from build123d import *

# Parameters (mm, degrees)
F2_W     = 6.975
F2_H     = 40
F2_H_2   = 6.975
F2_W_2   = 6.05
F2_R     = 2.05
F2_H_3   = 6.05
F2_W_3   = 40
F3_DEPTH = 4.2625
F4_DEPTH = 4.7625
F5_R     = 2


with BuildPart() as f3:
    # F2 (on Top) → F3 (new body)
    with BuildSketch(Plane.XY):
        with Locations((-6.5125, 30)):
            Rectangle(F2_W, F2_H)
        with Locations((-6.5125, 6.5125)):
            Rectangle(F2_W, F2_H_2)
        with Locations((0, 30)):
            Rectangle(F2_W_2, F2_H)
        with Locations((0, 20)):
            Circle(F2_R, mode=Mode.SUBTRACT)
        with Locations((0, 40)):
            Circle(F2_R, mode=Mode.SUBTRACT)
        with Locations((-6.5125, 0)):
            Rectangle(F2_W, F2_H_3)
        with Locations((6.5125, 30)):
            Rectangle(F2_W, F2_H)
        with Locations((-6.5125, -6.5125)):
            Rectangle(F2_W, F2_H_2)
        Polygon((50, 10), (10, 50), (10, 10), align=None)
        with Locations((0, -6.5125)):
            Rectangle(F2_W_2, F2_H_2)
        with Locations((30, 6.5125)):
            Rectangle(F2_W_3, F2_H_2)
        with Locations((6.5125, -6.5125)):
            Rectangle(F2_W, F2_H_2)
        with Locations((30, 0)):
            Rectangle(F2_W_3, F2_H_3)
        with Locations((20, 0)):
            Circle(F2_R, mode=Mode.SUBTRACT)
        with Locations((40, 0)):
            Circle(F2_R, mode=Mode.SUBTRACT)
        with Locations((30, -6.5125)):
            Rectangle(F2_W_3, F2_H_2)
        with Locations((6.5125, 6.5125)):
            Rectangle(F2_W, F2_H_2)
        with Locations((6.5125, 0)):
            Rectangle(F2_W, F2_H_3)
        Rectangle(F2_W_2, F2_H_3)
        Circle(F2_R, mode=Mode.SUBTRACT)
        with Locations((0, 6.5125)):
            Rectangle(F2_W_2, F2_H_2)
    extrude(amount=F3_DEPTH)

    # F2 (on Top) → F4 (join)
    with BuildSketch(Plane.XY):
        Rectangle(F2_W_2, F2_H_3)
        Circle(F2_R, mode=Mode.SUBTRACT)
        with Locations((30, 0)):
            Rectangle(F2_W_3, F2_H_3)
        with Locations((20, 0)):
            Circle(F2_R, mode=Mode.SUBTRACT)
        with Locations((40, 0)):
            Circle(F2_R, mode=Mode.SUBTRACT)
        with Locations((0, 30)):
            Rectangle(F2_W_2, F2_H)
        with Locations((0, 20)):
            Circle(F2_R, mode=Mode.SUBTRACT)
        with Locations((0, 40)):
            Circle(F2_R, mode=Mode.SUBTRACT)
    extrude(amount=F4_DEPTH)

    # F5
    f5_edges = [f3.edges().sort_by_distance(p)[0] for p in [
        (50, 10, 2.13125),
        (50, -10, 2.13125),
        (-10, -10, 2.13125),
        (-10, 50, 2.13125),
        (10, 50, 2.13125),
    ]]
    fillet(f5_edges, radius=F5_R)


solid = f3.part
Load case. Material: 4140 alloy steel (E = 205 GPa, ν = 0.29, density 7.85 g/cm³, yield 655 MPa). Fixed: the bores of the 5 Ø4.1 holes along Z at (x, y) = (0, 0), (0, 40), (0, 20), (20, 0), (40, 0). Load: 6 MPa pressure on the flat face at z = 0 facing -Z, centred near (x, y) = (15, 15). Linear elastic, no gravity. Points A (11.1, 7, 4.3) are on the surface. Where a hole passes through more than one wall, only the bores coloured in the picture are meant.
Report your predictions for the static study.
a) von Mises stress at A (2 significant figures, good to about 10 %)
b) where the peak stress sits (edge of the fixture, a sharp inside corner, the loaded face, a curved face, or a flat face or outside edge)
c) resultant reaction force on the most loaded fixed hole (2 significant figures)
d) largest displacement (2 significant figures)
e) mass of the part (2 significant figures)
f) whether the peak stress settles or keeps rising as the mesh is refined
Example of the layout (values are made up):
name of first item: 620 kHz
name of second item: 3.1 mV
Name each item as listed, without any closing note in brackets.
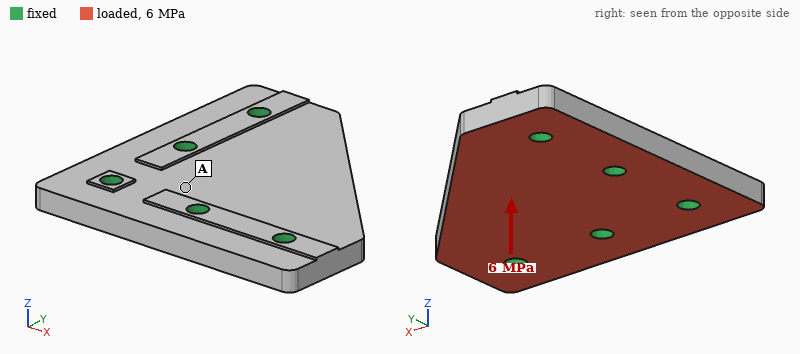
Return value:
von Mises stress at A: 100 MPa
where the peak stress sits: edge of the fixture
resultant reaction force on the most loaded fixed hole: 3.8 kN
largest displacement: 0.13 mm
mass of the part: 93 g
whether the peak stress settles or keeps rising as the mesh is refined: keeps rising
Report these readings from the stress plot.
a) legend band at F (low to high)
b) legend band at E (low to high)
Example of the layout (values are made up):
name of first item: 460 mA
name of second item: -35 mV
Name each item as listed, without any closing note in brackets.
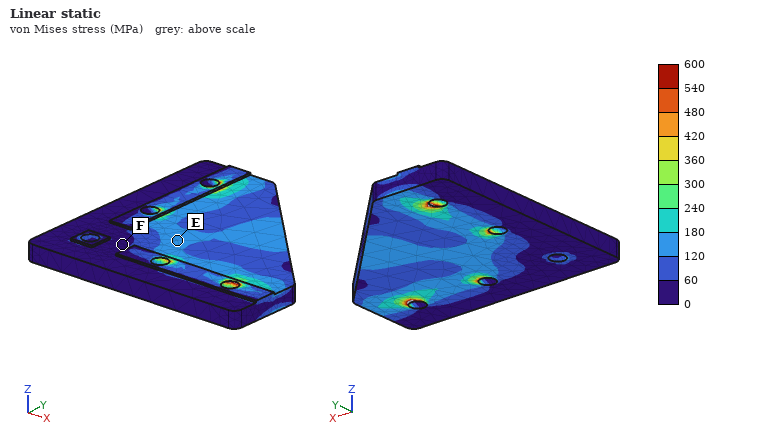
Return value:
legend band at F: 0 to 60 MPa
legend band at E: 120 to 180 MPa
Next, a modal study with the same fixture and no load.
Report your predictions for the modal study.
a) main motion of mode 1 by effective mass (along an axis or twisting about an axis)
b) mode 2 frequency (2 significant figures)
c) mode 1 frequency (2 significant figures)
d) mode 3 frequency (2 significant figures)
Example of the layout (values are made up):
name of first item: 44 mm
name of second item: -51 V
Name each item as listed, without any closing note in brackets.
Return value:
main motion of mode 1 by effective mass: along Z
mode 2 frequency: 16 kHz
mode 1 frequency: 8000 Hz
mode 3 frequency: 22 kHz
